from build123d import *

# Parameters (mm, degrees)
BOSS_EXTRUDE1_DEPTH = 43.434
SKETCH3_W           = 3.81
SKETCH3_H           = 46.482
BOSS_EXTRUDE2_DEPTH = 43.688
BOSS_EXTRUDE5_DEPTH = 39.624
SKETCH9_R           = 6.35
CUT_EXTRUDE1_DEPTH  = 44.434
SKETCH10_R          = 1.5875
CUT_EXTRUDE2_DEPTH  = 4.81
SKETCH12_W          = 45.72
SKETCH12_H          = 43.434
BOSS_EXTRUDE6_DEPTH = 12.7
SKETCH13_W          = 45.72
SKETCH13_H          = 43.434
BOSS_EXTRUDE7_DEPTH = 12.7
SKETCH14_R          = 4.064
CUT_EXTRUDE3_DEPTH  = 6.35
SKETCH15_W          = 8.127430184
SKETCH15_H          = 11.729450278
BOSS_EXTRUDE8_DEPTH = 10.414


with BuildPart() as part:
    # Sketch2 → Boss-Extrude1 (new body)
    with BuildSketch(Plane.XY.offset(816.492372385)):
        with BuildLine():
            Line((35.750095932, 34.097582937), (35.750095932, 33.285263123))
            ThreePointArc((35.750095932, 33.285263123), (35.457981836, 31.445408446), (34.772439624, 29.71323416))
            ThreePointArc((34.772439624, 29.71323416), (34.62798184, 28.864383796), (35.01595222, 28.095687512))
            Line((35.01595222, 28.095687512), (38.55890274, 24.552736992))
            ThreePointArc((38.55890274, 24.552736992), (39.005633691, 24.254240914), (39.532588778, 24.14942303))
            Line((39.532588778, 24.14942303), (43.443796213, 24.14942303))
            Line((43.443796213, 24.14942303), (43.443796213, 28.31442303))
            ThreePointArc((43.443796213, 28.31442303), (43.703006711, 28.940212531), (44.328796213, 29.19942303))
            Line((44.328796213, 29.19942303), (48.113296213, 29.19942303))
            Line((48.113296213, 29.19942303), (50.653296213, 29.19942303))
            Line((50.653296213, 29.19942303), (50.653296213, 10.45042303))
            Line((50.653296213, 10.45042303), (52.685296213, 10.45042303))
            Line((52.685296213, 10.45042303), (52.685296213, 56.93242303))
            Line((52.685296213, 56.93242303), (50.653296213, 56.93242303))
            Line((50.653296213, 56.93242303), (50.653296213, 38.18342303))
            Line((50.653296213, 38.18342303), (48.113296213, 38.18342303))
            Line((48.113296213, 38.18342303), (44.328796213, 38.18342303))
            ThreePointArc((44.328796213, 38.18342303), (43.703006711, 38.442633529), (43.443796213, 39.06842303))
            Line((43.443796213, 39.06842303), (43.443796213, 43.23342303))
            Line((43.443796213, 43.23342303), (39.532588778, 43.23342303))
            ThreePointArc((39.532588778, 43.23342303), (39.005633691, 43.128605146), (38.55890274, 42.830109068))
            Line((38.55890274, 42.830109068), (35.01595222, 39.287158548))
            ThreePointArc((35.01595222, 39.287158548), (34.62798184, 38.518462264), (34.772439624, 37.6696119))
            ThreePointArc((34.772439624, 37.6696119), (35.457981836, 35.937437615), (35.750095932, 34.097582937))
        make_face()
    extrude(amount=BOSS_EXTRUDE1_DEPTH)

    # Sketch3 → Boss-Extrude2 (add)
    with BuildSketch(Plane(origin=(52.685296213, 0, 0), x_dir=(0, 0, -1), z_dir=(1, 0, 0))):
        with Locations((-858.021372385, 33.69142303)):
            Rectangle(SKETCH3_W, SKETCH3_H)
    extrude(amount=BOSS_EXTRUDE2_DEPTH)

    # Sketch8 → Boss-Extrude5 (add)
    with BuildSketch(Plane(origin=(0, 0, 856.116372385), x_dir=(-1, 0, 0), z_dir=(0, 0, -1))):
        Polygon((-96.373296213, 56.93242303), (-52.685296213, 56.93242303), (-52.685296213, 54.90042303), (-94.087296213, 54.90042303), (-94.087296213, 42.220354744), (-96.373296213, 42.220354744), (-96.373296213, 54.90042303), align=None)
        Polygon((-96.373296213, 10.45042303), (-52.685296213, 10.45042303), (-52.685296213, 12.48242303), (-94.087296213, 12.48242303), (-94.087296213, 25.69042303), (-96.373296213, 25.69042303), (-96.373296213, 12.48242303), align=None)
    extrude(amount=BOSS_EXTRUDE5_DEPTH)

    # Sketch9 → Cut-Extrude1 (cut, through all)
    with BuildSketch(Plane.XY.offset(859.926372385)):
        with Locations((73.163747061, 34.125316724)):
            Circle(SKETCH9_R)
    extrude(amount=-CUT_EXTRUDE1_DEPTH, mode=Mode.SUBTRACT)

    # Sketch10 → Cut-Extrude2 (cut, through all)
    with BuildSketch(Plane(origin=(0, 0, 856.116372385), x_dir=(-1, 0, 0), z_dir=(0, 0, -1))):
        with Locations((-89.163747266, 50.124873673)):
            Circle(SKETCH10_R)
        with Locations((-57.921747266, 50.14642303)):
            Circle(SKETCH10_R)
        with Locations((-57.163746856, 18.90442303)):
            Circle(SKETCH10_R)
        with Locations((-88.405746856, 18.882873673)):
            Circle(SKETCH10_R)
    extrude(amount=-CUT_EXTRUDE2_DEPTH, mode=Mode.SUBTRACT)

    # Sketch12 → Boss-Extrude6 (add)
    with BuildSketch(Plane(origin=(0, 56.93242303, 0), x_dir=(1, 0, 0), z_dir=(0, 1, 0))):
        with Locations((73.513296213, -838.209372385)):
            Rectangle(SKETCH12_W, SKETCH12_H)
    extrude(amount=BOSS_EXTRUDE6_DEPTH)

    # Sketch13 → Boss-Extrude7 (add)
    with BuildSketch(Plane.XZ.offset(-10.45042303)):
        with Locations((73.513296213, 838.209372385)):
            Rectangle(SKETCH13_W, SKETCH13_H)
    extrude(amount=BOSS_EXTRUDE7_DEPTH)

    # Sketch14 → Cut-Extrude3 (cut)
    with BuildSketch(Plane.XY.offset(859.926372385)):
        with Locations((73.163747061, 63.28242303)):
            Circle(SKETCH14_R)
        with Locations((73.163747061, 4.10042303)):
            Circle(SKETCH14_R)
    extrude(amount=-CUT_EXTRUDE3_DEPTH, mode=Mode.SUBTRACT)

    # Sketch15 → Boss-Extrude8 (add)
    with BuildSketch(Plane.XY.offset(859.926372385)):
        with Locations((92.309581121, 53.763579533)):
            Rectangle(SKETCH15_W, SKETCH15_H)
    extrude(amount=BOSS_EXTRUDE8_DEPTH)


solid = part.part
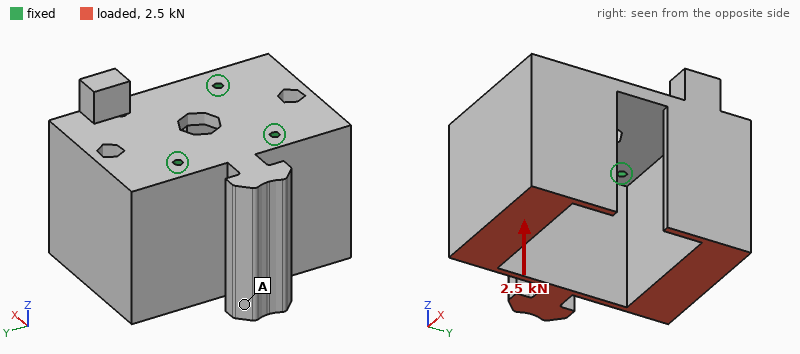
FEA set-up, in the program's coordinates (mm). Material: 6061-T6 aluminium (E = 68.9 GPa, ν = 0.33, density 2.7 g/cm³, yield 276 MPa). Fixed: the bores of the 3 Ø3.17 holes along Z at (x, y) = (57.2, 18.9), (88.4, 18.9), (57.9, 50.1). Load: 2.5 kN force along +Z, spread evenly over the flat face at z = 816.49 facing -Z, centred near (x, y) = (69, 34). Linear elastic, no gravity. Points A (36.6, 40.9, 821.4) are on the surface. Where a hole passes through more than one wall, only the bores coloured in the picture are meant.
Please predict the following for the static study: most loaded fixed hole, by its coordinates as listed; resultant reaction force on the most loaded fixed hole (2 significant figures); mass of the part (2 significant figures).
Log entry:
(57.9, 50.1)
1.2 kN
220 g
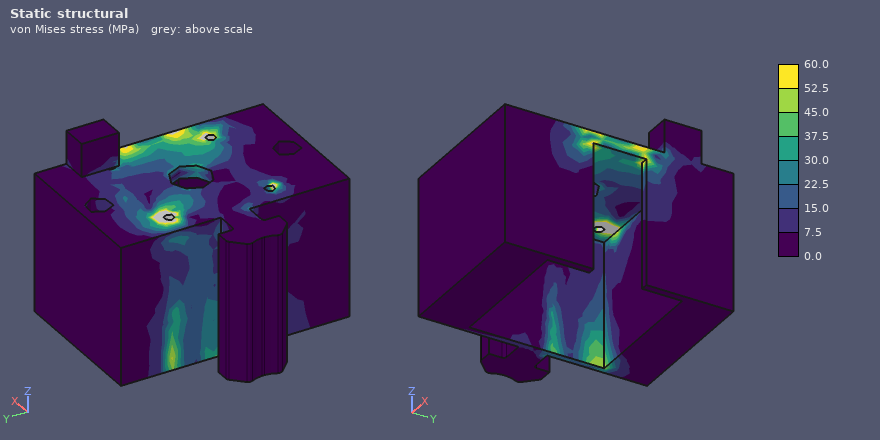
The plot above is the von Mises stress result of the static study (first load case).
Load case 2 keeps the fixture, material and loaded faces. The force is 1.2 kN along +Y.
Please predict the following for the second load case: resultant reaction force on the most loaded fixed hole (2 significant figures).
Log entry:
1.4 kN
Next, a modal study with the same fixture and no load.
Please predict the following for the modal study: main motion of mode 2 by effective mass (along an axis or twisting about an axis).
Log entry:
along Y
